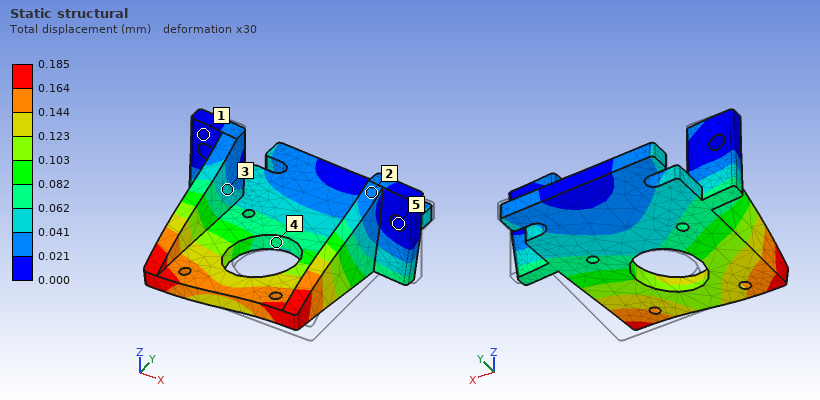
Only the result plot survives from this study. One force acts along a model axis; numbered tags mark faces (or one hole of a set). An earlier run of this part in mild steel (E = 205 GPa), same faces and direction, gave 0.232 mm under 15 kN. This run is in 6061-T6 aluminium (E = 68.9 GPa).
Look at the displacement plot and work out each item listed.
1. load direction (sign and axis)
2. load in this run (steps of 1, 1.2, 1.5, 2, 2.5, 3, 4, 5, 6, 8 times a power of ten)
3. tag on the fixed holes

-X
4 kN
5
